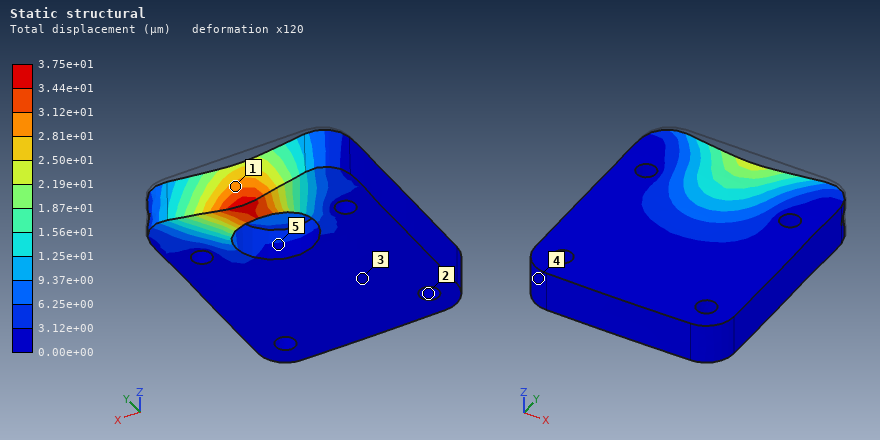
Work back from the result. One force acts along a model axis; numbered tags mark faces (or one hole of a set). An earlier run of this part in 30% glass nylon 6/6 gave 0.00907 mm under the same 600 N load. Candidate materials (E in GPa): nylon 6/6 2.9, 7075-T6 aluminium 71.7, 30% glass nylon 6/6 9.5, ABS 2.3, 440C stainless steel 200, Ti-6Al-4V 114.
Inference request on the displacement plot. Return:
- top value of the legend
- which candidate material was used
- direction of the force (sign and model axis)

3.75e+01 µm
ABS
-Y
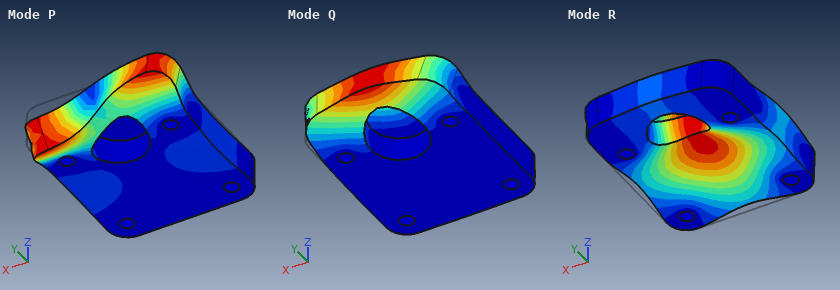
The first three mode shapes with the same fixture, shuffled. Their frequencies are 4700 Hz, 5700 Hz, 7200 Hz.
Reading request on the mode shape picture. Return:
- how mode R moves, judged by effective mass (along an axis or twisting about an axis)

along Z
